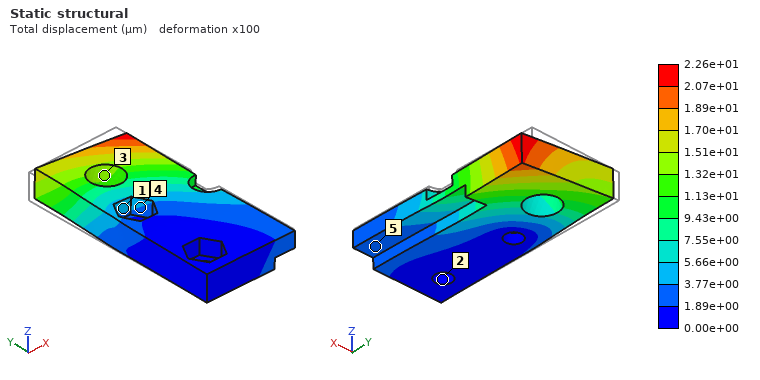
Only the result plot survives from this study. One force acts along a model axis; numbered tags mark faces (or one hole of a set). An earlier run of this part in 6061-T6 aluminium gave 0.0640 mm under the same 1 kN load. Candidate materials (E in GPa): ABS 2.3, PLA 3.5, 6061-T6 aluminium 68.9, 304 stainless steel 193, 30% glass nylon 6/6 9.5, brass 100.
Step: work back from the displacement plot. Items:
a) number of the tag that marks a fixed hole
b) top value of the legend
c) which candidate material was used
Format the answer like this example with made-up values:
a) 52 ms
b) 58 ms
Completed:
a) 2
b) 2.26e+01 µm
c) 304 stainless steel
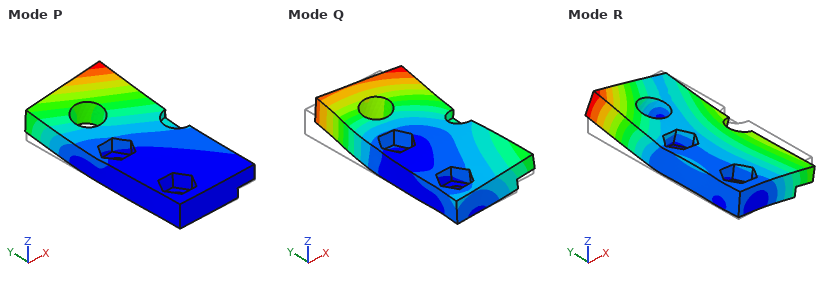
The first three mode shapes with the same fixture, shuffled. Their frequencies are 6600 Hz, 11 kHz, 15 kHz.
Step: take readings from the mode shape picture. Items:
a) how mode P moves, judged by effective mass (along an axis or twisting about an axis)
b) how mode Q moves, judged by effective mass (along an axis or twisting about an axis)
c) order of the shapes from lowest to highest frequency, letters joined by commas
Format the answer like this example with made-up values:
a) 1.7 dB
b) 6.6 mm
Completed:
a) along Z
b) along X
c) P, R, Q
